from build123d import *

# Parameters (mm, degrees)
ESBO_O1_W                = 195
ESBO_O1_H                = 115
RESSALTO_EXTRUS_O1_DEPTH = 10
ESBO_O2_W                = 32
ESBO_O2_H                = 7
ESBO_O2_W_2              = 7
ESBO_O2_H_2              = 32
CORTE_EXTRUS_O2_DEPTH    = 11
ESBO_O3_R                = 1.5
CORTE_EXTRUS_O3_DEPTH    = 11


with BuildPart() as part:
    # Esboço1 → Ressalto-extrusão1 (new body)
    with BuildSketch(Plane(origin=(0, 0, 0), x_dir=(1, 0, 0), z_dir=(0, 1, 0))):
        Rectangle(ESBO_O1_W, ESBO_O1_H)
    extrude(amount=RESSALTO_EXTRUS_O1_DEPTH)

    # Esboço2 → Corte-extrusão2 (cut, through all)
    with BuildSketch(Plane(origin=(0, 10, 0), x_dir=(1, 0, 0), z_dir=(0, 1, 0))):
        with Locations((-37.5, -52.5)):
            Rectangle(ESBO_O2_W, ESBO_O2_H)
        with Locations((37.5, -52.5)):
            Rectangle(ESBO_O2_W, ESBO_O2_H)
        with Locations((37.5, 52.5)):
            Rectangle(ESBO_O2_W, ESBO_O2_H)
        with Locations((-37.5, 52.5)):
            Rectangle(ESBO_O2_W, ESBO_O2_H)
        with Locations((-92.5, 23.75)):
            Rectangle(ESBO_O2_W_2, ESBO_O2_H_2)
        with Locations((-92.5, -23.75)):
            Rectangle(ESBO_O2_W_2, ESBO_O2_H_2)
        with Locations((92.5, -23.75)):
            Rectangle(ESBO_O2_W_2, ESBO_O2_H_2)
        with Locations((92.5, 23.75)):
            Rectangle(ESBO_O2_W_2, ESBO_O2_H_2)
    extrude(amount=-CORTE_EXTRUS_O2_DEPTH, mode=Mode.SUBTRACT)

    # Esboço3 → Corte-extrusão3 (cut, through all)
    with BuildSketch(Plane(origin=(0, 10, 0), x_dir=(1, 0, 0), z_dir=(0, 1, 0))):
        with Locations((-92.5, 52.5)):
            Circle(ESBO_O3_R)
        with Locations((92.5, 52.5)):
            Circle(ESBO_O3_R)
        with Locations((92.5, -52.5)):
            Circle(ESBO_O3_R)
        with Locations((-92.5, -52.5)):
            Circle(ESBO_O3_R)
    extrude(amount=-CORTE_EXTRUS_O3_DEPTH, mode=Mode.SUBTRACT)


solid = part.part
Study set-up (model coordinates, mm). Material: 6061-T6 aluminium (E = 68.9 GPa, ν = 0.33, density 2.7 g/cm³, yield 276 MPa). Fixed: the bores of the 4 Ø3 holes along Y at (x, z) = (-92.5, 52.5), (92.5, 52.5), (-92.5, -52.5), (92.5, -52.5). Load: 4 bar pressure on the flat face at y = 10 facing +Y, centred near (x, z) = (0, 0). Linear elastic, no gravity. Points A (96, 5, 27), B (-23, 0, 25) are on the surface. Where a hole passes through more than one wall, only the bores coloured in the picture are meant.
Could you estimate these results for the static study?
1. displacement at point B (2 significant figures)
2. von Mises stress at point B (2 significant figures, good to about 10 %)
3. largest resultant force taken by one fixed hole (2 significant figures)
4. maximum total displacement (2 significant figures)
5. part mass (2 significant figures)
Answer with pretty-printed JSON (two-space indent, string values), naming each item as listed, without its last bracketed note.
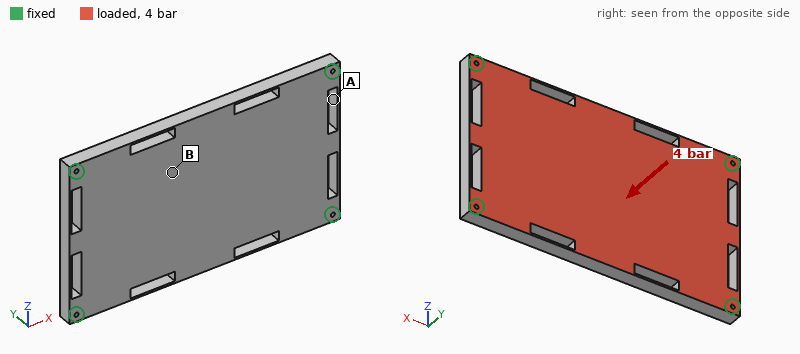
{
  "displacement at point B": "0.41 mm",
  "von Mises stress at point B": "42 MPa",
  "largest resultant force taken by one fixed hole": "2.1 kN",
  "maximum total displacement": "0.45 mm",
  "part mass": "560 g"
}
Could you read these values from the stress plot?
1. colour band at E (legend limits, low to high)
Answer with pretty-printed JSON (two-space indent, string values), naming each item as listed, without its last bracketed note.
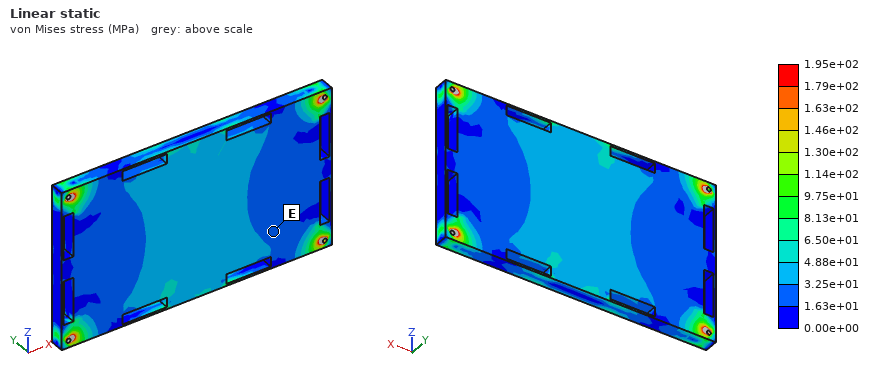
{
  "colour band at E": "1.63e+01 to 3.25e+01 MPa"
}
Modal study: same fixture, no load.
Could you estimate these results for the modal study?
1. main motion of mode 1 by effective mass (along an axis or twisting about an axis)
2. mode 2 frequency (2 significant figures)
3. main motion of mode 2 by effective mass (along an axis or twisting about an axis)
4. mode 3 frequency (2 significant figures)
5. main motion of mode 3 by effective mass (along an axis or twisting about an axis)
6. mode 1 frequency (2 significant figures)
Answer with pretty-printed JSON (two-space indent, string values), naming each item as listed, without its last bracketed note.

{
  "main motion of mode 1 by effective mass": "along Y",
  "mode 2 frequency": "2000 Hz",
  "main motion of mode 2 by effective mass": "twisting about X",
  "mode 3 frequency": "2800 Hz",
  "main motion of mode 3 by effective mass": "twisting about Z",
  "mode 1 frequency": "1000 Hz"
}
